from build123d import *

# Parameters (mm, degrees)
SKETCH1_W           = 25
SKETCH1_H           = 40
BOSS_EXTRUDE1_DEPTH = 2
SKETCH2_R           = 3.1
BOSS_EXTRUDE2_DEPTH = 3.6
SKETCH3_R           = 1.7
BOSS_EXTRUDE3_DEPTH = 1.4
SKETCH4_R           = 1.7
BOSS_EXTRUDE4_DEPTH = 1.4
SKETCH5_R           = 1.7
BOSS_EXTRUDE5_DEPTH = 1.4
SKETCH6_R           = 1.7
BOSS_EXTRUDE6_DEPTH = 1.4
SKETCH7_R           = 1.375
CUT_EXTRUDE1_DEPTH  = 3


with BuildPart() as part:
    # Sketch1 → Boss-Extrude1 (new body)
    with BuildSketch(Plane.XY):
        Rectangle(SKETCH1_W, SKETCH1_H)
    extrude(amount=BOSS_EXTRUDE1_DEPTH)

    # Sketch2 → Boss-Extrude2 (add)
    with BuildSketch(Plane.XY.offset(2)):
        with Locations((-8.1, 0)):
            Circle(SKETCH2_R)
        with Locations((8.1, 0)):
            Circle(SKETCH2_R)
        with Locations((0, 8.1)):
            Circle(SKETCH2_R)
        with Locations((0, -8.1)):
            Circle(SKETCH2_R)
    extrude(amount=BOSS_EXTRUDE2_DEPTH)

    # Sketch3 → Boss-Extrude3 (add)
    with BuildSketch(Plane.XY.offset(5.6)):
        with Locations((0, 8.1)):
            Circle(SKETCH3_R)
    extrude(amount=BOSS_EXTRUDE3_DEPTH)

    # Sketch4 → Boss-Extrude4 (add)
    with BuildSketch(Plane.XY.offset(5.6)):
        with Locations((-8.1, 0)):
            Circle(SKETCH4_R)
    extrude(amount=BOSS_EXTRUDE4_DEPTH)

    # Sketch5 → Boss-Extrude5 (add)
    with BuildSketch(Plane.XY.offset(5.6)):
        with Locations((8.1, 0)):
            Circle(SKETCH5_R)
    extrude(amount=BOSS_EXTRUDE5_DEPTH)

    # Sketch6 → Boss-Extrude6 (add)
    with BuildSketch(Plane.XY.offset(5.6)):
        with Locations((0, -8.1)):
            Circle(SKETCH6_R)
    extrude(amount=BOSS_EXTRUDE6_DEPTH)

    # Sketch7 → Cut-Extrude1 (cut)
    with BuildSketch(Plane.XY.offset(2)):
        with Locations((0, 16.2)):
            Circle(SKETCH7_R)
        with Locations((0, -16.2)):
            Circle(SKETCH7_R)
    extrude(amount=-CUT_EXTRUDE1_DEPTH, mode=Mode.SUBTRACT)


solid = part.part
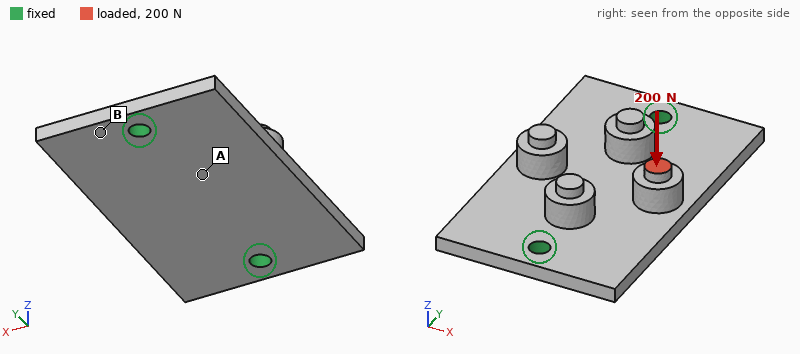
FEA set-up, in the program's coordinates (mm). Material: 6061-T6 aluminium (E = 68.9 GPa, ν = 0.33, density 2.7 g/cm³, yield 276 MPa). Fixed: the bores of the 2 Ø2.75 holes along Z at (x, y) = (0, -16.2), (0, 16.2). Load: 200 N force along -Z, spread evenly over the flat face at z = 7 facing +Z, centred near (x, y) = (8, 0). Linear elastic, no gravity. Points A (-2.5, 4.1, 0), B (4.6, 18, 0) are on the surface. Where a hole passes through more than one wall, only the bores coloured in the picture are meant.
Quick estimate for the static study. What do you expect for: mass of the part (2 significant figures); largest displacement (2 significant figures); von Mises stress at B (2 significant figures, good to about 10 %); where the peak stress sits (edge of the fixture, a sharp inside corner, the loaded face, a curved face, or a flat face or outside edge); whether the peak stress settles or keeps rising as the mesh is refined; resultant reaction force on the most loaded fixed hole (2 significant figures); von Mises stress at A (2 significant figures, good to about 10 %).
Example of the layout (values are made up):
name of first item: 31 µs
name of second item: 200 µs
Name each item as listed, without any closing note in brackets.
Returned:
mass of the part: 6.6 g
largest displacement: 0.11 mm
von Mises stress at B: 60 MPa
where the peak stress sits: edge of the fixture
whether the peak stress settles or keeps rising as the mesh is refined: keeps rising
resultant reaction force on the most loaded fixed hole: 100 N
von Mises stress at A: 26 MPa
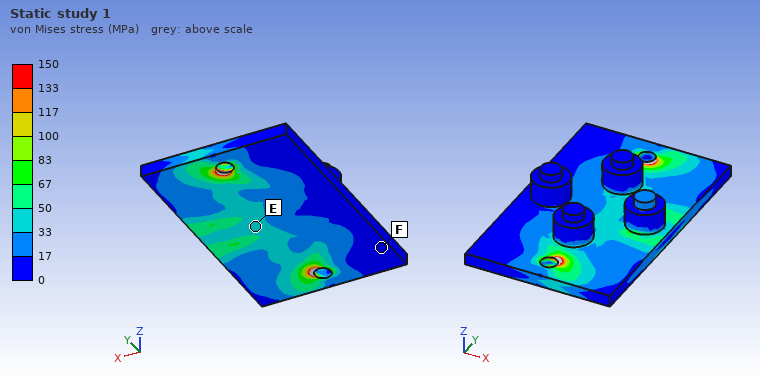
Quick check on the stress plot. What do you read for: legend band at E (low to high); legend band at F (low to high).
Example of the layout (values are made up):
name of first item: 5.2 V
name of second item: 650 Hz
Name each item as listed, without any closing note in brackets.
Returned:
legend band at E: 33 to 50 MPa
legend band at F: 0 to 17 MPa
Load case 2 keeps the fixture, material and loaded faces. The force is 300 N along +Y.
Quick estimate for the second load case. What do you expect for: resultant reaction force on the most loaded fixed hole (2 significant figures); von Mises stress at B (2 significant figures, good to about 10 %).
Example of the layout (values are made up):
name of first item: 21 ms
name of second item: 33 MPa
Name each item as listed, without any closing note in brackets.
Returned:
resultant reaction force on the most loaded fixed hole: 180 N
von Mises stress at B: 26 MPa
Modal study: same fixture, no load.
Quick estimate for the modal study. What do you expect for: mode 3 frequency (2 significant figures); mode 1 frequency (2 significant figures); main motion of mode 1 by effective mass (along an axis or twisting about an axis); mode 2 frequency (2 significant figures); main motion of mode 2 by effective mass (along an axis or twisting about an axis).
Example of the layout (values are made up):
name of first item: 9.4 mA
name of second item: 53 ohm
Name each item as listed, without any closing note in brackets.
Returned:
mode 3 frequency: 13 kHz
mode 1 frequency: 5800 Hz
main motion of mode 1 by effective mass: twisting about Y
mode 2 frequency: 6800 Hz
main motion of mode 2 by effective mass: along Z
